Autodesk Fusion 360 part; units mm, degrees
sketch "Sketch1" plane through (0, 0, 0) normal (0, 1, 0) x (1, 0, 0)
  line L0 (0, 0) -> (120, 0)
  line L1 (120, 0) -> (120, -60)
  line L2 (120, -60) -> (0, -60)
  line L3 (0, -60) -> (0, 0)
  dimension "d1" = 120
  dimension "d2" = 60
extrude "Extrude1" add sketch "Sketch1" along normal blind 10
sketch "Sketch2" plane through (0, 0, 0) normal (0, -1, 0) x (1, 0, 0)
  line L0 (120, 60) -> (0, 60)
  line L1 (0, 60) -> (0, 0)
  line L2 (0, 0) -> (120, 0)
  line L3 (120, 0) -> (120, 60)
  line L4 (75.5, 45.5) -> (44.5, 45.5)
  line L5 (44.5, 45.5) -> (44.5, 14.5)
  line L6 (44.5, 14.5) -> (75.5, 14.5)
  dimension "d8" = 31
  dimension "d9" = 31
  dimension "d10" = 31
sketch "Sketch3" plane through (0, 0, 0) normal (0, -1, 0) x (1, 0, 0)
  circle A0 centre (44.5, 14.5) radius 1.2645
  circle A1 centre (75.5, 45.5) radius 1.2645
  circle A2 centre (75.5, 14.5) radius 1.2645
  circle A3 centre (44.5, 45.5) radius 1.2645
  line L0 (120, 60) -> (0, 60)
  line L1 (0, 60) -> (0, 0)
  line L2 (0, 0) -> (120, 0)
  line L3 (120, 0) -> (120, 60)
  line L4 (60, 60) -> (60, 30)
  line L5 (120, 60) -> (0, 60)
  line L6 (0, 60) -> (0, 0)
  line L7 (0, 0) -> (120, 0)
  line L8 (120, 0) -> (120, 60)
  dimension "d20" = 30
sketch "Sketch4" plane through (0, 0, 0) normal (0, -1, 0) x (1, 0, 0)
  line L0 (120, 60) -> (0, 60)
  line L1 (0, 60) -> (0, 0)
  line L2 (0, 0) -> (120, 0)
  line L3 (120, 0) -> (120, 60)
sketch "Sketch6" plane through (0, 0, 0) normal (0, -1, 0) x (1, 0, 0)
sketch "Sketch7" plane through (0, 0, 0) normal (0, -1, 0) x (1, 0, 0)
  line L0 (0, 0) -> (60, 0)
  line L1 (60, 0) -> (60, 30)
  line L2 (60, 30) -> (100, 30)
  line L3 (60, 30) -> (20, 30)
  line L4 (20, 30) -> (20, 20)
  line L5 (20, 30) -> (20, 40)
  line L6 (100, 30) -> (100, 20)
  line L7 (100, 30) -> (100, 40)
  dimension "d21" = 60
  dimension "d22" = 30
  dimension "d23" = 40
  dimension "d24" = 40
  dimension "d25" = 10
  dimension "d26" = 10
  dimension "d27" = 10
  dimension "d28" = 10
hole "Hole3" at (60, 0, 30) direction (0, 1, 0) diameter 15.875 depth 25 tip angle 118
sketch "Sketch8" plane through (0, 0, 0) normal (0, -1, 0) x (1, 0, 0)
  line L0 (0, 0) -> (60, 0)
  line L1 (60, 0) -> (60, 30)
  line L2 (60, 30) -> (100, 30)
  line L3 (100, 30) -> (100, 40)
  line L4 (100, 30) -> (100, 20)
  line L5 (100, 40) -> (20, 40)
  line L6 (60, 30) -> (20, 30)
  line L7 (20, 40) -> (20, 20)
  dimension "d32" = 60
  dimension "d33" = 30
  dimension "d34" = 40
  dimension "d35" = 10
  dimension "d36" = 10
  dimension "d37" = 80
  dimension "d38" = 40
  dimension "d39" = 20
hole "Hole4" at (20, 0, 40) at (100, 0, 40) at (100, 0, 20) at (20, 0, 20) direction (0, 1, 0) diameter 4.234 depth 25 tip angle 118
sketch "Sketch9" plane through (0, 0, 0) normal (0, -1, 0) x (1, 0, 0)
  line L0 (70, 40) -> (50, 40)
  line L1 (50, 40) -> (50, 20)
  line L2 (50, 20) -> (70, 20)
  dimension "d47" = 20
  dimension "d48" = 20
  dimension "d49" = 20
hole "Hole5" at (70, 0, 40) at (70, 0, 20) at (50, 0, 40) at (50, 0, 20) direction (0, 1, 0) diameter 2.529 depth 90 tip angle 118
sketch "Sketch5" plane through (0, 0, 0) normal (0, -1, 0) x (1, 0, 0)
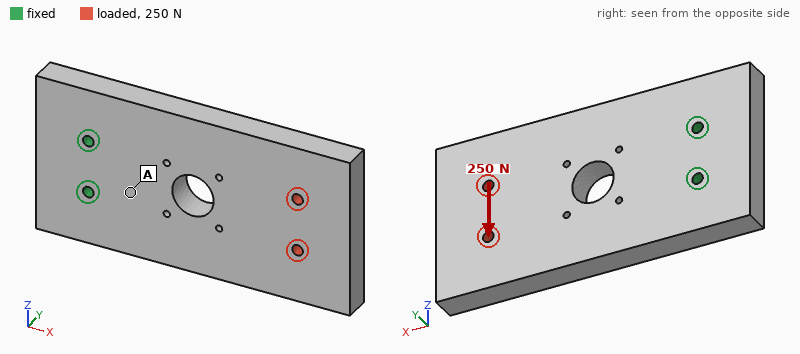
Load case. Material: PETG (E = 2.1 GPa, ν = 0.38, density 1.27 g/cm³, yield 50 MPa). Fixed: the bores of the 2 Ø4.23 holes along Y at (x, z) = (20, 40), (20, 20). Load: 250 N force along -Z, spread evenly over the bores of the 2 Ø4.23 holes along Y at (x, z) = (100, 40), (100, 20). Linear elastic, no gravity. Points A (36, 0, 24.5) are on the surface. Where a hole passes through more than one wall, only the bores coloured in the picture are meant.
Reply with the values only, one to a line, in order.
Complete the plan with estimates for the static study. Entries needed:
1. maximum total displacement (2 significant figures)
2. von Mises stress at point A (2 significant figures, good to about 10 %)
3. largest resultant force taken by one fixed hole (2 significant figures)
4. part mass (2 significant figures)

0.48 mm
2.5 MPa
890 N
88 g
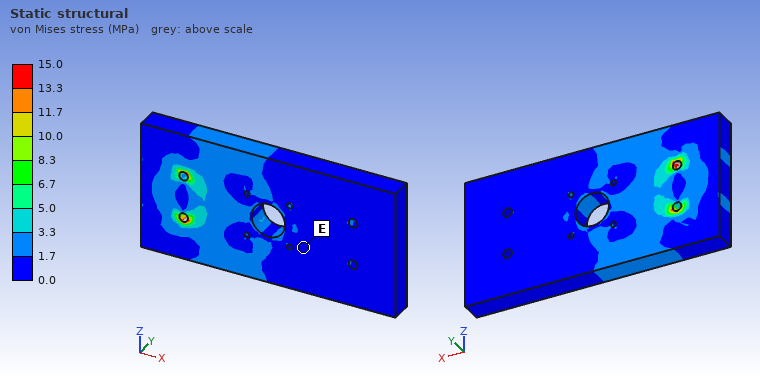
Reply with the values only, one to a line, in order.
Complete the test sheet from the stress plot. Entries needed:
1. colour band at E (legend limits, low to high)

0.0 to 1.7 MPa
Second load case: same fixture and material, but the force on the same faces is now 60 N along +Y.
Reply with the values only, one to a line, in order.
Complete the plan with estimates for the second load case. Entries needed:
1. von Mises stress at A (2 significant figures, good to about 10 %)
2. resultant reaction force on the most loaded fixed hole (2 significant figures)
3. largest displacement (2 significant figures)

3.5 MPa
30 N
1.6 mm
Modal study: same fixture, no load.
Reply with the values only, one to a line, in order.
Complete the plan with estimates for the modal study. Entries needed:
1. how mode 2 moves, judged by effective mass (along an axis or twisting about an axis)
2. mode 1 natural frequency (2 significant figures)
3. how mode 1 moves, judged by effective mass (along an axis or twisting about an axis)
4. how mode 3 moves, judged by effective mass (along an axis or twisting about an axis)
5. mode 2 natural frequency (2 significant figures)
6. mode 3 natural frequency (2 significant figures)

twisting about X
190 Hz
along Y
along Z
620 Hz
650 Hz
